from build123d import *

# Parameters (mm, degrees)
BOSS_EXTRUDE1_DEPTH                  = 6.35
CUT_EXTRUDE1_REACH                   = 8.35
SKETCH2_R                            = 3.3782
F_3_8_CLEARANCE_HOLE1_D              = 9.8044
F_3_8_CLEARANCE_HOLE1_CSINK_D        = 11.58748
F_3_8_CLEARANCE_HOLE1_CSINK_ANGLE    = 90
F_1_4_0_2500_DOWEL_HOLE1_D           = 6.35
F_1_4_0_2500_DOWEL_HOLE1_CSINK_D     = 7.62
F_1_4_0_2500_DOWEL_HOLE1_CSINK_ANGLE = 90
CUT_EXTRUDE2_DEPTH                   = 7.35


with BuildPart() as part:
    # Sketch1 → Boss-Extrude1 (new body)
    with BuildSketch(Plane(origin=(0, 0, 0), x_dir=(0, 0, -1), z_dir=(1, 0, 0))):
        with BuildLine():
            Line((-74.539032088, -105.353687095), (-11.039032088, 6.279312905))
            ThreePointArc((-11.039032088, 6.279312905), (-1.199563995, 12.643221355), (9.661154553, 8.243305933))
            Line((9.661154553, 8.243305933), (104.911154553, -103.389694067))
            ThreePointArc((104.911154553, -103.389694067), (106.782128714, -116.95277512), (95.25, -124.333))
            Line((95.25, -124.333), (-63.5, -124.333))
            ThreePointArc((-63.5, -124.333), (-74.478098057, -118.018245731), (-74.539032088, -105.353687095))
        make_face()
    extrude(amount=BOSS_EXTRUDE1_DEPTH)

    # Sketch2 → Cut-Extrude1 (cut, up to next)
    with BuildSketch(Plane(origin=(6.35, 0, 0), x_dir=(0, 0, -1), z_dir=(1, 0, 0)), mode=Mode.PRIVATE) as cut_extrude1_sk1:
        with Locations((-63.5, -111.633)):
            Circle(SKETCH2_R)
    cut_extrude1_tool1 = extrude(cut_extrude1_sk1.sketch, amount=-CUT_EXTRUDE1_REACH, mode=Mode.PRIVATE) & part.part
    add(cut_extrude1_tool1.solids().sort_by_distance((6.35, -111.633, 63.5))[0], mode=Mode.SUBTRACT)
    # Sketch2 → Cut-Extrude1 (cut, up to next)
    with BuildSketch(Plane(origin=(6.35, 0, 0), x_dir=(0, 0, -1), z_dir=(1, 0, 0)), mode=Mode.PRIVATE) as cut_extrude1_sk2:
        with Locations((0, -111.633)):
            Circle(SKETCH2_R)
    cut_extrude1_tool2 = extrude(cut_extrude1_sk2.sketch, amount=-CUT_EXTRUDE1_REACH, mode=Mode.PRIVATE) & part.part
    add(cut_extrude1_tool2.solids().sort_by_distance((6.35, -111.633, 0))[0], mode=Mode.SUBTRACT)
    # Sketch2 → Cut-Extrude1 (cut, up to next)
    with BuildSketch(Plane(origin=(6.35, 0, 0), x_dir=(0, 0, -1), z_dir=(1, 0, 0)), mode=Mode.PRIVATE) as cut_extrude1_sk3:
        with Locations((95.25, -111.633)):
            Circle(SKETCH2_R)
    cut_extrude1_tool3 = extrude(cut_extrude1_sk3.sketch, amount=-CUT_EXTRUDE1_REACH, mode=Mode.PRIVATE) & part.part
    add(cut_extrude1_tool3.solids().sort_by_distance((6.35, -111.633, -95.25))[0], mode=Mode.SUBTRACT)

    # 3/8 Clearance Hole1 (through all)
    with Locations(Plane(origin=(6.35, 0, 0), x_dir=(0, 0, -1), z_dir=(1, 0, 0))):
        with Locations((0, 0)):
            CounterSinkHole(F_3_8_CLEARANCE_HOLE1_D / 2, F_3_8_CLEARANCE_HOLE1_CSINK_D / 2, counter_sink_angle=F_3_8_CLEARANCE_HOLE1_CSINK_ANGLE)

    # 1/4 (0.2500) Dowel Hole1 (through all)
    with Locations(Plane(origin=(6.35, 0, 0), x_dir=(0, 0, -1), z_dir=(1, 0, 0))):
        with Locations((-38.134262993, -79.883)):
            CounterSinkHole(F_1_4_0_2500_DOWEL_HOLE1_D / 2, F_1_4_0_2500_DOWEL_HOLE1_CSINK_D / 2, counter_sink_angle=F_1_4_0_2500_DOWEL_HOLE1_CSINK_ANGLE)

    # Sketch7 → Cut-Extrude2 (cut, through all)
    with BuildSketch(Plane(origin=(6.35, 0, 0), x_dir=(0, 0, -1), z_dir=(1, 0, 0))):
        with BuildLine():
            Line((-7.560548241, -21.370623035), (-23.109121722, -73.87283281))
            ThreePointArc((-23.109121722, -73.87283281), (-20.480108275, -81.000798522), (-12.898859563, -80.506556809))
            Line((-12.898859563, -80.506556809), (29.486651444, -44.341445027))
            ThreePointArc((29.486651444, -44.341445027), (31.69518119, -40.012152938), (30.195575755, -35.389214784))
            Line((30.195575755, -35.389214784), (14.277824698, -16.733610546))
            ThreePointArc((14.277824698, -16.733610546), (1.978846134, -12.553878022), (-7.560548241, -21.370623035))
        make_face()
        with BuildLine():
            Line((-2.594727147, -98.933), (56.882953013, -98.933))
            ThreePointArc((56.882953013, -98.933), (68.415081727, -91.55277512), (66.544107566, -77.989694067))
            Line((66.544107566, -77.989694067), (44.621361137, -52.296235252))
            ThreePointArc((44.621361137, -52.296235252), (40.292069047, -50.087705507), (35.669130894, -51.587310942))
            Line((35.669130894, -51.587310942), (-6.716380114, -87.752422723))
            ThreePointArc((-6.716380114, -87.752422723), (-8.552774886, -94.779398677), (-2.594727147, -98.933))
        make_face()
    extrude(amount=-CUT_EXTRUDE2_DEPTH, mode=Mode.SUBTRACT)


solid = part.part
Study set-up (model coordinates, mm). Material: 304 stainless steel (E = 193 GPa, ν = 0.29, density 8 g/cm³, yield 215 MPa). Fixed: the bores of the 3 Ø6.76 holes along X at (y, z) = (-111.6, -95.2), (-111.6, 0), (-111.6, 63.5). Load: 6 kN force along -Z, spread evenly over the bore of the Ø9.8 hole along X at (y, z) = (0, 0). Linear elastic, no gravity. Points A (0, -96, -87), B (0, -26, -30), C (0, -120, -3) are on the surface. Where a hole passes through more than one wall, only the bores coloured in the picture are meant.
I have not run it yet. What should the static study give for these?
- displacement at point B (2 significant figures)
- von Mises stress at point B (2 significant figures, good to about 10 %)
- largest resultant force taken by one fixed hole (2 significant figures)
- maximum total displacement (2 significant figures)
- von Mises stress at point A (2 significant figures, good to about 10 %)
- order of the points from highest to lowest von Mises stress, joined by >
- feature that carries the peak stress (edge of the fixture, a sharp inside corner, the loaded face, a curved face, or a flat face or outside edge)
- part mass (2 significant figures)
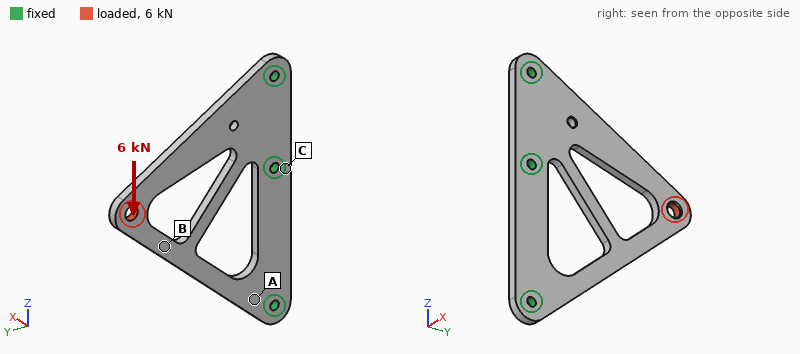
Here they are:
44 µm
71 MPa
4.9 kN
68 µm
38 MPa
B > A > C
the loaded face
520 g
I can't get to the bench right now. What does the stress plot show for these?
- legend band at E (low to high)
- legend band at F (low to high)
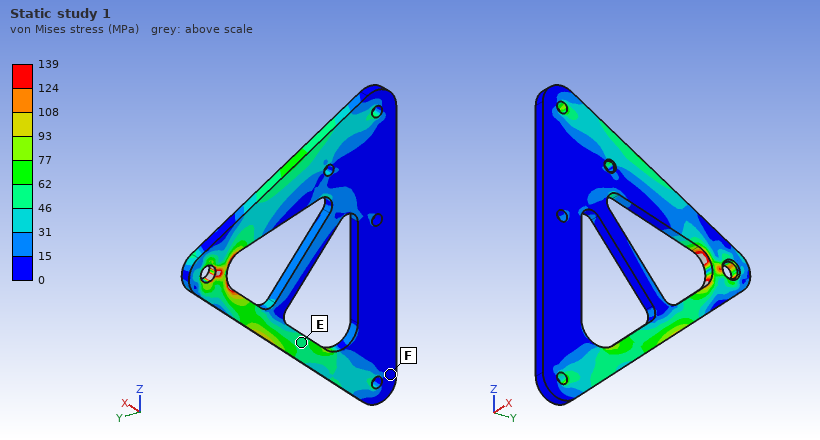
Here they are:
46 to 62 MPa
0 to 15 MPa
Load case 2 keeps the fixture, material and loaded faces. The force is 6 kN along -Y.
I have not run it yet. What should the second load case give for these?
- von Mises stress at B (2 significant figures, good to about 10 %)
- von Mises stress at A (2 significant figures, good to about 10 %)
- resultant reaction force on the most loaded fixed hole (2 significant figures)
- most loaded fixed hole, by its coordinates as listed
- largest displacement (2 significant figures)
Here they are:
45 MPa
26 MPa
3.5 kN
(-111.6, 63.5)
0.11 mm
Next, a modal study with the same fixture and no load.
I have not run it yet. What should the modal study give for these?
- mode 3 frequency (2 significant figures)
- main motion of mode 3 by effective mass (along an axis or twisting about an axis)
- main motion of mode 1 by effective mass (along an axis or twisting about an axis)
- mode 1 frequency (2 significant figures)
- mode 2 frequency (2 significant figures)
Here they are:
1900 Hz
along X
along X
430 Hz
1300 Hz
